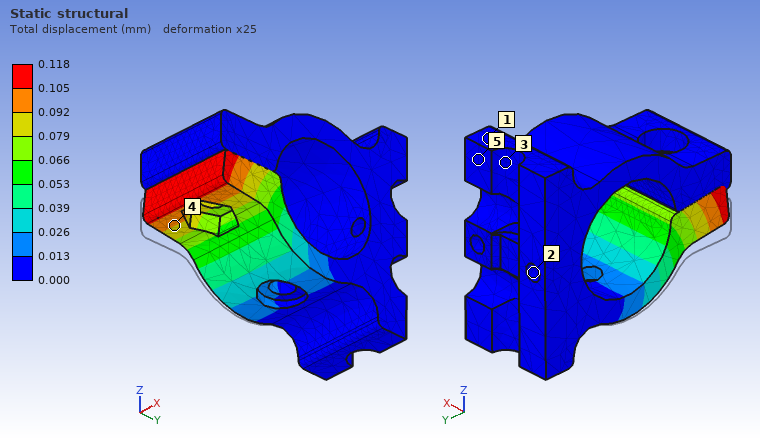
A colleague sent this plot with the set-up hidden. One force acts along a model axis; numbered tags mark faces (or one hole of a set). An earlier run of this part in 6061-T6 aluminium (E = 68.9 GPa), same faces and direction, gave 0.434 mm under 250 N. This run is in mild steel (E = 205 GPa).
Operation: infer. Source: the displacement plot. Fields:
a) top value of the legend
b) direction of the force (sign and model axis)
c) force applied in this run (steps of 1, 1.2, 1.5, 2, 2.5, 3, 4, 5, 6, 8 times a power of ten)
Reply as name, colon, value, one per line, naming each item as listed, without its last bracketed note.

top value of the legend: 0.118 mm
direction of the force: +Z
force applied in this run: 200 N
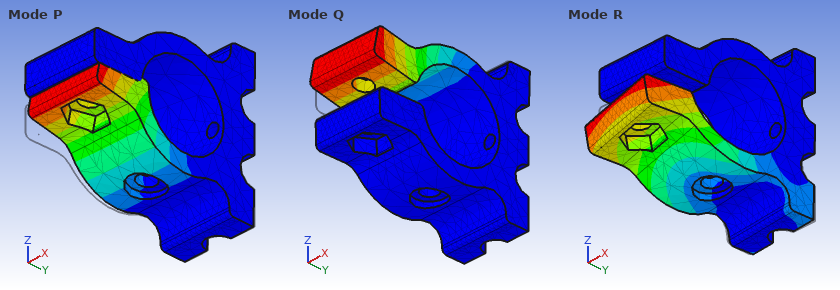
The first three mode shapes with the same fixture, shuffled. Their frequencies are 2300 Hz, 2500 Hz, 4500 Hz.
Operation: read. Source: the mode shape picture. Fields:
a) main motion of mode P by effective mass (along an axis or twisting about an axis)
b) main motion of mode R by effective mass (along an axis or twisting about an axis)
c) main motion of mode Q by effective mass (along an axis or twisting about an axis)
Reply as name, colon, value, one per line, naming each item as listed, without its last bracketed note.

main motion of mode P by effective mass: along Z
main motion of mode R by effective mass: along X
main motion of mode Q by effective mass: along Z
